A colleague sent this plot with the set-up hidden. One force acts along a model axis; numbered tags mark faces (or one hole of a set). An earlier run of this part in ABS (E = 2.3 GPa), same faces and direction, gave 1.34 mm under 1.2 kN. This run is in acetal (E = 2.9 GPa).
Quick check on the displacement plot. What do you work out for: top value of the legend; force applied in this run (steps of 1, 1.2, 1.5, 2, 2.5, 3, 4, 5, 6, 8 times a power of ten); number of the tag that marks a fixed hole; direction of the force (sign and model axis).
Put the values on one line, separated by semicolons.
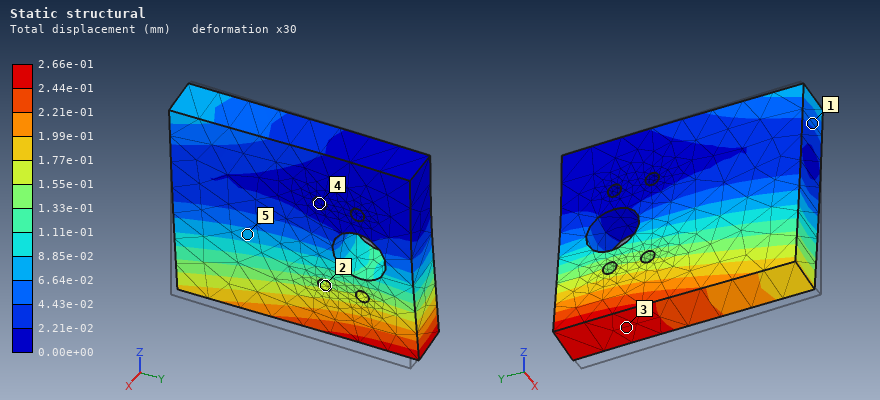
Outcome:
2.66e-01 mm; 300 N; 4; -X
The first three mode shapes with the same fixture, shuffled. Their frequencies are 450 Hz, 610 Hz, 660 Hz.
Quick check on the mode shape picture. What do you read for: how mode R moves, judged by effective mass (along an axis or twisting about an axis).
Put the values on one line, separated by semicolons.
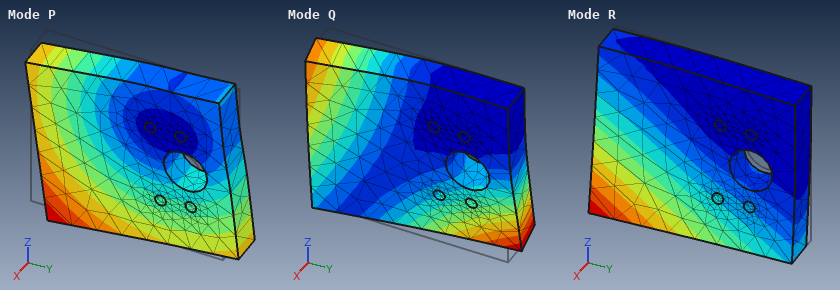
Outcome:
along X
